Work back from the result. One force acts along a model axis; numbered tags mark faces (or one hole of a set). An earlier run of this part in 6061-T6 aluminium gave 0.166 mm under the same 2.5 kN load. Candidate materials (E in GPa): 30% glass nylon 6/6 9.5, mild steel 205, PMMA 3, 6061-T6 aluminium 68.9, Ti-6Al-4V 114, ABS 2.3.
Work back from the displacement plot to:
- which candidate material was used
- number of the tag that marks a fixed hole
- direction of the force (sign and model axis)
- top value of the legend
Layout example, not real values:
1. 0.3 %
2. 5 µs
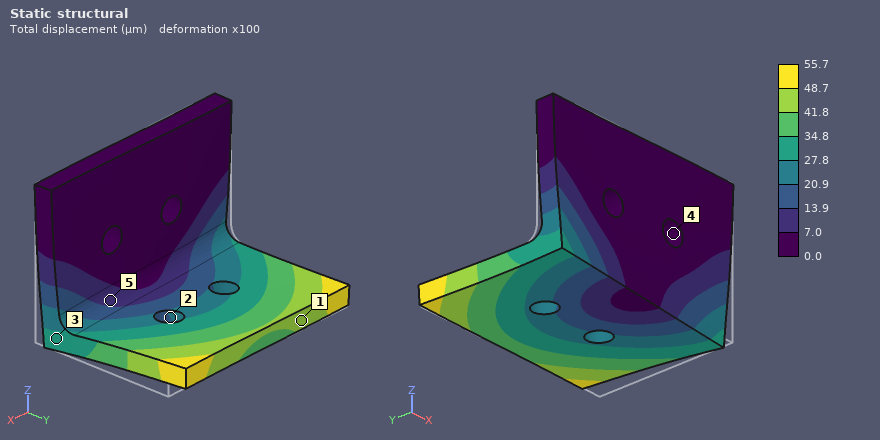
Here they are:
1. mild steel
2. 4
3. -X
4. 55.7 µm
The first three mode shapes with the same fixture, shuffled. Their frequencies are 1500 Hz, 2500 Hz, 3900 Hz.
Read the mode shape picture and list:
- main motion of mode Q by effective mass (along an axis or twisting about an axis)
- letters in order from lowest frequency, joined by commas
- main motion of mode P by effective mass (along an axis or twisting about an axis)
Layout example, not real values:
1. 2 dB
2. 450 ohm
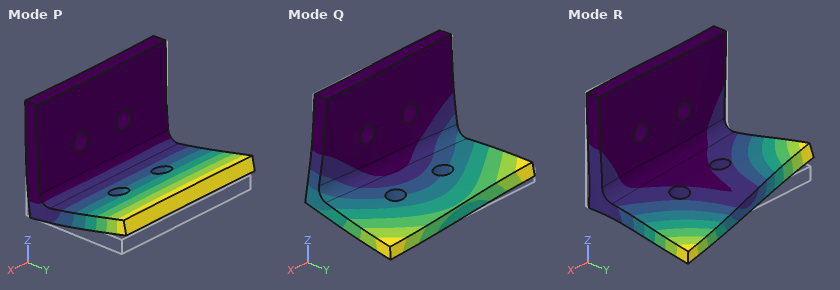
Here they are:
1. along X
2. P, Q, R
3. along Z
